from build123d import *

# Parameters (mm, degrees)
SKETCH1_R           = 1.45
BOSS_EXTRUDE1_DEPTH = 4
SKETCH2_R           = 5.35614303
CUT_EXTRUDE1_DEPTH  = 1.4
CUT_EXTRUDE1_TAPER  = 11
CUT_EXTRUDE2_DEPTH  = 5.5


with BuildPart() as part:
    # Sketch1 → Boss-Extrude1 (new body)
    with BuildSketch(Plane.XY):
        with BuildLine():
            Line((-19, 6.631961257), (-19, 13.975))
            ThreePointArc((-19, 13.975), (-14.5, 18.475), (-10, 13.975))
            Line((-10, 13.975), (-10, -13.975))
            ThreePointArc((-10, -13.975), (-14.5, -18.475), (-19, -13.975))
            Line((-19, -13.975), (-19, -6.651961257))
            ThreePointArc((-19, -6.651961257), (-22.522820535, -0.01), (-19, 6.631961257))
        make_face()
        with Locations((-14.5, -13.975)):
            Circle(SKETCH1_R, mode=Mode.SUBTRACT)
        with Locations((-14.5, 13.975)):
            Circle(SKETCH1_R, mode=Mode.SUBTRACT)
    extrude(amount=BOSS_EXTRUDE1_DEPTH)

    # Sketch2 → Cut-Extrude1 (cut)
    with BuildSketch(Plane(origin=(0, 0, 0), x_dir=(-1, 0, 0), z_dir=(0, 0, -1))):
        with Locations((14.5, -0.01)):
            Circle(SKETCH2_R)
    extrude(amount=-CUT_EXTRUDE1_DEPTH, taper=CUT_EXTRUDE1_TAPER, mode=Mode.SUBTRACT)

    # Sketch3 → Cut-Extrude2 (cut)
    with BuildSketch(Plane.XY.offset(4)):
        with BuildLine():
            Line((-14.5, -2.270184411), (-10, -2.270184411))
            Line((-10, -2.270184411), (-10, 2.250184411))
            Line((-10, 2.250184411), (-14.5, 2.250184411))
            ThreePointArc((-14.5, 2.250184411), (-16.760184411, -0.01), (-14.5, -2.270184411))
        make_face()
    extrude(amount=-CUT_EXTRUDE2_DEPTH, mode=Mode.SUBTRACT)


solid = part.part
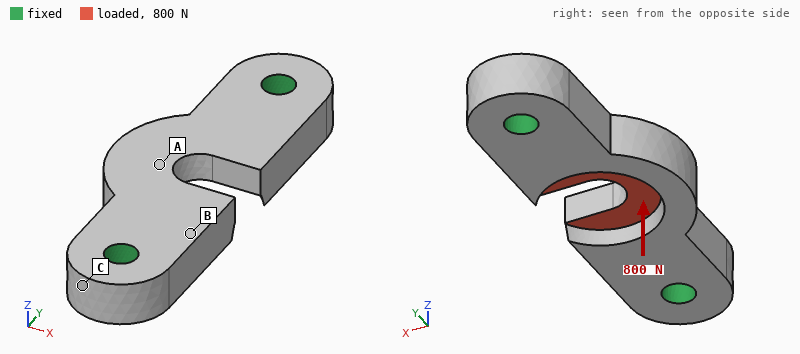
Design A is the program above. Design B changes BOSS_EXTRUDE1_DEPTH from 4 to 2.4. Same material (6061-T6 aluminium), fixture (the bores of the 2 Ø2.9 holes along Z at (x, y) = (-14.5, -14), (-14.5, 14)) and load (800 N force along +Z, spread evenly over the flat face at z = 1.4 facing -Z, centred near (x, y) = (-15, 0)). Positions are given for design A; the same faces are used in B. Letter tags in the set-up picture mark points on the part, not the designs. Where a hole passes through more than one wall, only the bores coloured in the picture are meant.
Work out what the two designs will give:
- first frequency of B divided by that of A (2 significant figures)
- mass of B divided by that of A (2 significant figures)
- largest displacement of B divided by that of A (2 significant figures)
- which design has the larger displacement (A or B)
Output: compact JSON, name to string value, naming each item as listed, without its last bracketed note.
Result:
{"first frequency of B divided by that of A": "0.71", "mass of B divided by that of A": "0.57", "largest displacement of B divided by that of A": "4.3", "which design has the larger displacement": "B"}
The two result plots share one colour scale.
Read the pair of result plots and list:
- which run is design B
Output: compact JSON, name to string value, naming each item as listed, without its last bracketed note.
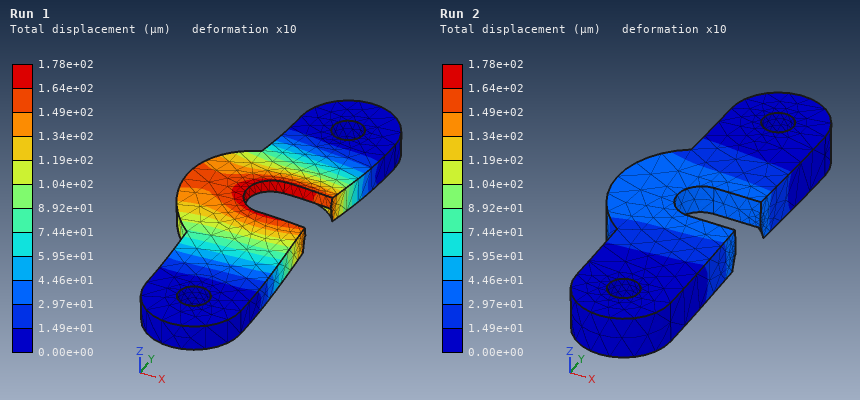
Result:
{"which run is design B": "Run 1"}
